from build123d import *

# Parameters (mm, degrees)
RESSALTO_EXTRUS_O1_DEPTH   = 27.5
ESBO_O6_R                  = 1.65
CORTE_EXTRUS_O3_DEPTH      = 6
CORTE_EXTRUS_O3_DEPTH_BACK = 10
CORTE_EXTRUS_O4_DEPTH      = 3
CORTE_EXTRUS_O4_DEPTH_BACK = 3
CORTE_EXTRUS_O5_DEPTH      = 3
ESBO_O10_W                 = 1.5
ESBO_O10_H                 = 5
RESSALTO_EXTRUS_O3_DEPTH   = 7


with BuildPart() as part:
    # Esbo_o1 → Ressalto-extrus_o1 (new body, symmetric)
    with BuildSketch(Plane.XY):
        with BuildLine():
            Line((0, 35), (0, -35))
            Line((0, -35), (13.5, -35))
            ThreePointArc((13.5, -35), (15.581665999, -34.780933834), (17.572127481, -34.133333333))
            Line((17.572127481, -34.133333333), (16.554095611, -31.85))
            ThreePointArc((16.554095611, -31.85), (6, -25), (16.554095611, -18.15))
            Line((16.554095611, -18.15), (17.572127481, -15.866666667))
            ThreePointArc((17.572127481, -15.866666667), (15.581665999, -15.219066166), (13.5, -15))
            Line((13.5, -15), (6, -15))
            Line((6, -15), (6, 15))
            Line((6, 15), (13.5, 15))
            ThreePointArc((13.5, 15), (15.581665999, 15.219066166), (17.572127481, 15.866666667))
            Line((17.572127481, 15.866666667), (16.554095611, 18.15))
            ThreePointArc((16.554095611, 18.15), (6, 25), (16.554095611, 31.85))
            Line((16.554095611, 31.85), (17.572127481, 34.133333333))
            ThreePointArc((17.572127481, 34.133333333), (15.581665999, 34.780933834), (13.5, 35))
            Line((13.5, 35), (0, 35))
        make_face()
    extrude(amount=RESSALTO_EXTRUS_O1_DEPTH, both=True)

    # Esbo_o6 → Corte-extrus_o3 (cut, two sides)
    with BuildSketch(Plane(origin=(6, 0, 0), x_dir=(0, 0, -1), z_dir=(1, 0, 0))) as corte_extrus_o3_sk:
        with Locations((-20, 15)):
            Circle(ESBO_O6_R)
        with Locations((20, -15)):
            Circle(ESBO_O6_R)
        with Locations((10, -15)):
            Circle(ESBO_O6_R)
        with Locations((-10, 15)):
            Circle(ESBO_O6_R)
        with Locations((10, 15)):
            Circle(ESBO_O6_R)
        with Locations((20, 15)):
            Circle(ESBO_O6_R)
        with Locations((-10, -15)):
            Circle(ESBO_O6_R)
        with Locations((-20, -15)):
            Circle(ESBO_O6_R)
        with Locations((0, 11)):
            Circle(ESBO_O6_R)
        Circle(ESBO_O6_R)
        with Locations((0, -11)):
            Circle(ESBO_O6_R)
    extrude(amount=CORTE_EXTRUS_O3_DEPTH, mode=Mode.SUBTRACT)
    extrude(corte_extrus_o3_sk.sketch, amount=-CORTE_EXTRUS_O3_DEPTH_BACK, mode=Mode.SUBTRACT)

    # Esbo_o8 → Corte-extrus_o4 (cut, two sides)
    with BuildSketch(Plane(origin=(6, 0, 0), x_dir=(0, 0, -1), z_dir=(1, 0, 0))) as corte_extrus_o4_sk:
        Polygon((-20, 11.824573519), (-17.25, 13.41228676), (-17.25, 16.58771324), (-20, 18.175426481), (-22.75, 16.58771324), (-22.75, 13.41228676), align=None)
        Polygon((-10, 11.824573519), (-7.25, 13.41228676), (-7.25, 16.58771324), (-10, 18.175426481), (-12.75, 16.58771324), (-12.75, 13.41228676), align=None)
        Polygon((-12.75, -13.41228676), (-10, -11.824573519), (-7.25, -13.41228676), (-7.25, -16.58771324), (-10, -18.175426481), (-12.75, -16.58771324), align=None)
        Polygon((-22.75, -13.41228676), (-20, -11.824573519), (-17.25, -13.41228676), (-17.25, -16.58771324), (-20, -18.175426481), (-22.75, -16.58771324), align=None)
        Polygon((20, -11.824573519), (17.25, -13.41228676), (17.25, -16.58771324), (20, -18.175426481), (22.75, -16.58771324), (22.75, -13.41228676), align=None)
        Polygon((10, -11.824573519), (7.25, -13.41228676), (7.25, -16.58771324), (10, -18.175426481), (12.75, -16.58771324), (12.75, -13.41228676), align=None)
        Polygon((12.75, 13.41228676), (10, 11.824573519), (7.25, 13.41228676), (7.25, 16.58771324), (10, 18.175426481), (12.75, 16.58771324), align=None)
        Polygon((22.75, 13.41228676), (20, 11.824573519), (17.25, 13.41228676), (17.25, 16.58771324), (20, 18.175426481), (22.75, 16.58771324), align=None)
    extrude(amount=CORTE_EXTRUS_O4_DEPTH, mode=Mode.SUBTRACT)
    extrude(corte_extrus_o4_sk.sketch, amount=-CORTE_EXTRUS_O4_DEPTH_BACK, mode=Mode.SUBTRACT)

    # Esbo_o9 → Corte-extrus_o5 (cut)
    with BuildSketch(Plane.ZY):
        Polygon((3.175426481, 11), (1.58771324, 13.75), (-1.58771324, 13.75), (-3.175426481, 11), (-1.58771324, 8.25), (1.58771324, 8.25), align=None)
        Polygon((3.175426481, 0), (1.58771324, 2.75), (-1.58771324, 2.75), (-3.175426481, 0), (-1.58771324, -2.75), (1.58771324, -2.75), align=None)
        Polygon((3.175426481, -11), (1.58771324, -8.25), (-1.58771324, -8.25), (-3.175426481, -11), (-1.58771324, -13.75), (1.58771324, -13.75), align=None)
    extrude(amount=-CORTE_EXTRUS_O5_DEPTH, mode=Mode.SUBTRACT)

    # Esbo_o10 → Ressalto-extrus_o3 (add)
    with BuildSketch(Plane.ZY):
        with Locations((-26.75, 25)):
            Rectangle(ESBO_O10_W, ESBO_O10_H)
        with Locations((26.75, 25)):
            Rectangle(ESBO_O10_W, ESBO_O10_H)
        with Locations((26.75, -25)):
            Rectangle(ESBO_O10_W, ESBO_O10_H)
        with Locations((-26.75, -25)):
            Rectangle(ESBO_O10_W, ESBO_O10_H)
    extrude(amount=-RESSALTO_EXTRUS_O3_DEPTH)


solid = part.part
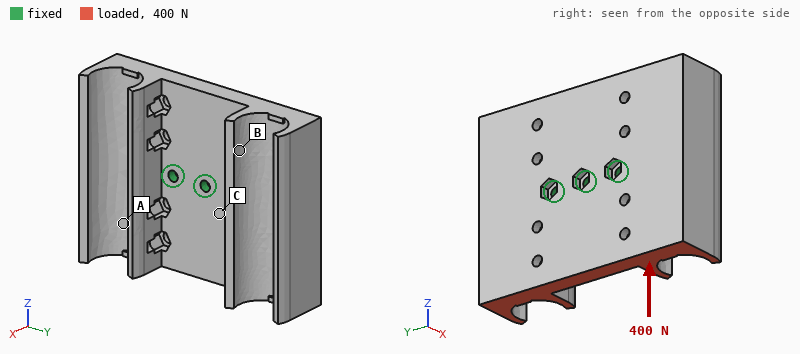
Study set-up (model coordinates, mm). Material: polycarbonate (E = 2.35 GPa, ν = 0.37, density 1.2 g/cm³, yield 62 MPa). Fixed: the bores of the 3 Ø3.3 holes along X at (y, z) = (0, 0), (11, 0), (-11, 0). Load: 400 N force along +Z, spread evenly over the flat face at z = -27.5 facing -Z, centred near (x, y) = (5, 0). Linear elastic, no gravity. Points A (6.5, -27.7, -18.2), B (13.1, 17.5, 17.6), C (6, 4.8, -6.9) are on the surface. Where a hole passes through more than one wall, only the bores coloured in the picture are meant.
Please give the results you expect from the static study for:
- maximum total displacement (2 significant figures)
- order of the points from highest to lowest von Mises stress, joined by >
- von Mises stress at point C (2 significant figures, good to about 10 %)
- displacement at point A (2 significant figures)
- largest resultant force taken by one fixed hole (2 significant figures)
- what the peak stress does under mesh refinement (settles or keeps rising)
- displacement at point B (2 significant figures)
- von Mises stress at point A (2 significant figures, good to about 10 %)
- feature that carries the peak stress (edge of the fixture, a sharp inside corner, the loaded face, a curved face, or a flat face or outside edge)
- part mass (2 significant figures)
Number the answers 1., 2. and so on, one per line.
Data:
1. 88 µm
2. C > A > B
3. 1.7 MPa
4. 48 µm
5. 150 N
6. keeps rising
7. 42 µm
8. 0.93 MPa
9. edge of the fixture
10. 36 g
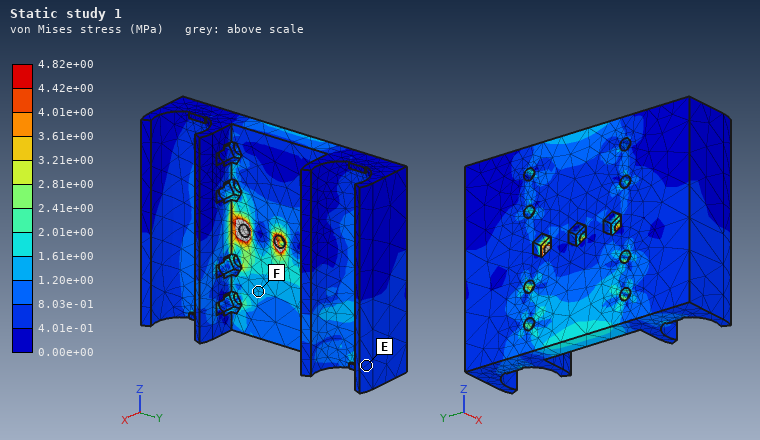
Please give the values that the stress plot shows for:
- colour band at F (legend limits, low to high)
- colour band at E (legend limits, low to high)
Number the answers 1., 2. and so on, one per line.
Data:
1. 1.20e+00 to 1.61e+00 MPa
2. 4.01e-01 to 8.03e-01 MPa
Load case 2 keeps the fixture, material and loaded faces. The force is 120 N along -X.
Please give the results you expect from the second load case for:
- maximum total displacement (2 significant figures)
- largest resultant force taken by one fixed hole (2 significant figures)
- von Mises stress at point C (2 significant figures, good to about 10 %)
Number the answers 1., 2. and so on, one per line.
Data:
1. 0.78 mm
2. 74 N
3. 4.8 MPa
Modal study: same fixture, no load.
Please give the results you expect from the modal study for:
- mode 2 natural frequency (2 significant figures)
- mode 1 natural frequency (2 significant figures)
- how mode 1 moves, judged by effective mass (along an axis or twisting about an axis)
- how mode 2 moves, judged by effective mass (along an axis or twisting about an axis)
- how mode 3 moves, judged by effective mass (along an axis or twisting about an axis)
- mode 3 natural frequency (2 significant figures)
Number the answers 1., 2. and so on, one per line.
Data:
1. 980 Hz
2. 640 Hz
3. twisting about Y
4. twisting about Z
5. along X
6. 1100 Hz
